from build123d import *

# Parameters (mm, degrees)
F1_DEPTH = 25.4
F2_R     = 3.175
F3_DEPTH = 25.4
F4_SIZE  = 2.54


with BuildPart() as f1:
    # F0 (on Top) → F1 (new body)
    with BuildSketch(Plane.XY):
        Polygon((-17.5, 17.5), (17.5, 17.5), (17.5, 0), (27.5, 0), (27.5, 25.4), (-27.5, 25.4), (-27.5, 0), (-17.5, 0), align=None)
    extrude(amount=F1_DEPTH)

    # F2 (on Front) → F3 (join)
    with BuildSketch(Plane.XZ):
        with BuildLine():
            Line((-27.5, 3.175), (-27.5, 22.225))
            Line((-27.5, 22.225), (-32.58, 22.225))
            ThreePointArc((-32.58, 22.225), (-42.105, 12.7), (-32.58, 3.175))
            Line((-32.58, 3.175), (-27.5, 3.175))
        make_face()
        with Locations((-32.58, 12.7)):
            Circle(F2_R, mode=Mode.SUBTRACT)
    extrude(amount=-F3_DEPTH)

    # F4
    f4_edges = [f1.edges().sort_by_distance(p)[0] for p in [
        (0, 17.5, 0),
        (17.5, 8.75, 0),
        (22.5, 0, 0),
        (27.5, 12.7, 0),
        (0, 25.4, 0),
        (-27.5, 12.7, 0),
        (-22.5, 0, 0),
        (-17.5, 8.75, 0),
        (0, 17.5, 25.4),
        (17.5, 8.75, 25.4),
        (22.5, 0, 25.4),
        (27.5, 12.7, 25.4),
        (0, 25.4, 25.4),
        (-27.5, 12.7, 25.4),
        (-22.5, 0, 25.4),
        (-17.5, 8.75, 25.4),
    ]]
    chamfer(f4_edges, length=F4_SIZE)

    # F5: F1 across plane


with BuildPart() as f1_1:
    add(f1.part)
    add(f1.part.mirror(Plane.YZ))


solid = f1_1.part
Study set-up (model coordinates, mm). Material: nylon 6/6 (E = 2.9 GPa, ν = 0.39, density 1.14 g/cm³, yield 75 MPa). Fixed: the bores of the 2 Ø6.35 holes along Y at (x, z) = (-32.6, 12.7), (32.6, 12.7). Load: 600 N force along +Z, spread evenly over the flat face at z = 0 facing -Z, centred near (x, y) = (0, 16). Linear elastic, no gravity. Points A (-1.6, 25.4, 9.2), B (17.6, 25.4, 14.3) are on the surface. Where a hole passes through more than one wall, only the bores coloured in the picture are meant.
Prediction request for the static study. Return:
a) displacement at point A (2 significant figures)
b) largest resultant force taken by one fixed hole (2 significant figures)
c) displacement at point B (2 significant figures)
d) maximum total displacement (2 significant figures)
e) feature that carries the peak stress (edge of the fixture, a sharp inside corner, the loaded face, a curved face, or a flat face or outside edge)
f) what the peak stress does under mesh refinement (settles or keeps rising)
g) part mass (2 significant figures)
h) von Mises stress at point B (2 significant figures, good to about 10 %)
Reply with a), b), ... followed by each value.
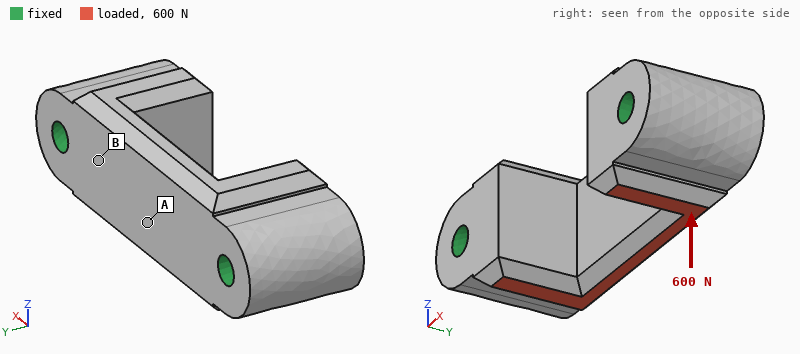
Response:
a) 36 µm
b) 300 N
c) 22 µm
d) 37 µm
e) edge of the fixture
f) keeps rising
g) 33 g
h) 1.5 MPa
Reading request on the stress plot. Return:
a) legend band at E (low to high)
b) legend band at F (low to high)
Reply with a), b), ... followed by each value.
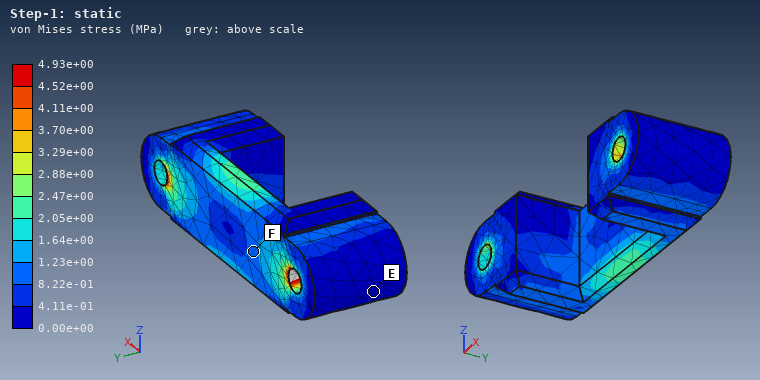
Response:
a) 0.00e+00 to 4.11e-01 MPa
b) 8.22e-01 to 1.23e+00 MPa
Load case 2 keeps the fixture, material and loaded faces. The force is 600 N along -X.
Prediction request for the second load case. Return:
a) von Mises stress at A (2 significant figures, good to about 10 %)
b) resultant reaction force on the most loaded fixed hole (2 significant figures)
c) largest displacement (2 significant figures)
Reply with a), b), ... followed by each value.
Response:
a) 0.89 MPa
b) 310 N
c) 20 µm
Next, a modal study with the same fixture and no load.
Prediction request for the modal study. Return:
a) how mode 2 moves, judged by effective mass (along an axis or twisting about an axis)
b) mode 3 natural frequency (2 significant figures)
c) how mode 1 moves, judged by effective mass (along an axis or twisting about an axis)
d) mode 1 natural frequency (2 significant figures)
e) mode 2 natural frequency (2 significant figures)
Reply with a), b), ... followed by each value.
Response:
a) along Y
b) 7500 Hz
c) along Z
d) 5100 Hz
e) 5300 Hz
